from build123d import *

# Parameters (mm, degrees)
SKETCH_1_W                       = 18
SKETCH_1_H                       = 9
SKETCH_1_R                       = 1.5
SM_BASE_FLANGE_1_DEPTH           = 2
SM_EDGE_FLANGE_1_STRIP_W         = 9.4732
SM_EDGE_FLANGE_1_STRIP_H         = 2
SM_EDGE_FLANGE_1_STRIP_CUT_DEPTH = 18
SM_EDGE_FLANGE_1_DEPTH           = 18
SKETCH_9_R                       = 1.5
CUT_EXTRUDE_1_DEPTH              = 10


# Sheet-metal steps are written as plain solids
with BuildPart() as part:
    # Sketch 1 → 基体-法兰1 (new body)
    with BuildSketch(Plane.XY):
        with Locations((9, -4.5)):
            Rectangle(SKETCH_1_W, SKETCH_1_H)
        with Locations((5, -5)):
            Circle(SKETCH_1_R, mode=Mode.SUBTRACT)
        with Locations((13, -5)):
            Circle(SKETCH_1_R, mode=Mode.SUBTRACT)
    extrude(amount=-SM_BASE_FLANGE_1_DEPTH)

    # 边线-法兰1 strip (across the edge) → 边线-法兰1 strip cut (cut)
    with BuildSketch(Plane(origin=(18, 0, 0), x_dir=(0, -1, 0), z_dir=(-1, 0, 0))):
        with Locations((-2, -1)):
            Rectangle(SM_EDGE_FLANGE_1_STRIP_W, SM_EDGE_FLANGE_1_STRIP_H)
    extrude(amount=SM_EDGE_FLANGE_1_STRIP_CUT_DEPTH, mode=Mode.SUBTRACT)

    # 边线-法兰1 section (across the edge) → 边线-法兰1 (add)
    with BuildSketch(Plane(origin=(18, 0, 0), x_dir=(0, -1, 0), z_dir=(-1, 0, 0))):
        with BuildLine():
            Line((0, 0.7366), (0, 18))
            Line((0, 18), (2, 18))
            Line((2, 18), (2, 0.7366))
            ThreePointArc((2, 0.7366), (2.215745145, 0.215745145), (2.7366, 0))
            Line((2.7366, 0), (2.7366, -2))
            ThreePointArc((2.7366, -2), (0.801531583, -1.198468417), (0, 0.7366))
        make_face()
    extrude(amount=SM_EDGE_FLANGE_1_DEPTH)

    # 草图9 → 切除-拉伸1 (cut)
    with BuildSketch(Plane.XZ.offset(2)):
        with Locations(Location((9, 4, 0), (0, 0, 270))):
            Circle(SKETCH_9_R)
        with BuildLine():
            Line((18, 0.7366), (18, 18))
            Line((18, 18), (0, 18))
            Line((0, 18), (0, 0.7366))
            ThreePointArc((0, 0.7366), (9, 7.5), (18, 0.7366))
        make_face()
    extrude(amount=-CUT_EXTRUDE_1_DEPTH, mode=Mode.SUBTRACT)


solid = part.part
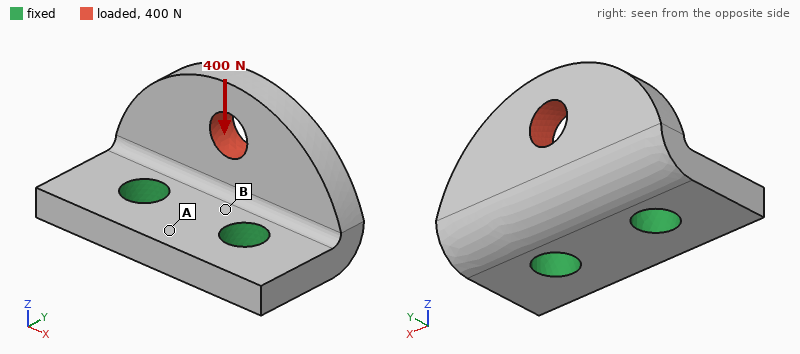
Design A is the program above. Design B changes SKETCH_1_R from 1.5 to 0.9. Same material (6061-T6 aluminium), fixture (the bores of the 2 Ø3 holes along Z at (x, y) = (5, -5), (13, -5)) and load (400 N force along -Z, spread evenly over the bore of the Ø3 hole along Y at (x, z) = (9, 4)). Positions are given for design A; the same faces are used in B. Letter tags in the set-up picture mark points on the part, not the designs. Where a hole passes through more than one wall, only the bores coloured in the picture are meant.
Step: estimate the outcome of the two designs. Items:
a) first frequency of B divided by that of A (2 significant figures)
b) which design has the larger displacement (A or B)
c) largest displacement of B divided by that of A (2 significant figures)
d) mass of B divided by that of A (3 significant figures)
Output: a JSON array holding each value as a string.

["0.88", "B", "1.5", "1.04"]
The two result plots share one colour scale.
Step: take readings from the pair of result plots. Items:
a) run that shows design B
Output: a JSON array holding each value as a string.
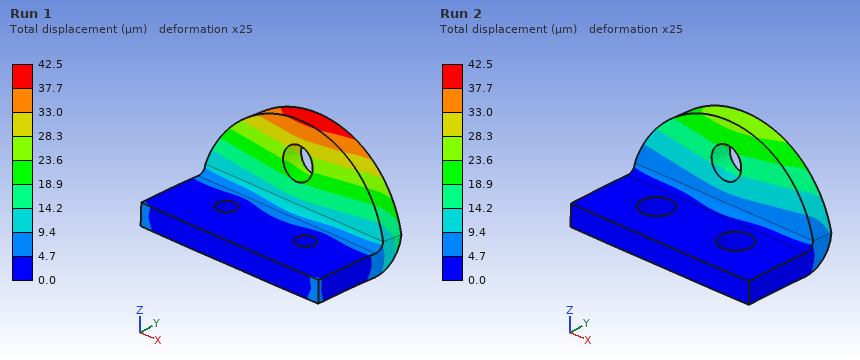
["Run 1"]
